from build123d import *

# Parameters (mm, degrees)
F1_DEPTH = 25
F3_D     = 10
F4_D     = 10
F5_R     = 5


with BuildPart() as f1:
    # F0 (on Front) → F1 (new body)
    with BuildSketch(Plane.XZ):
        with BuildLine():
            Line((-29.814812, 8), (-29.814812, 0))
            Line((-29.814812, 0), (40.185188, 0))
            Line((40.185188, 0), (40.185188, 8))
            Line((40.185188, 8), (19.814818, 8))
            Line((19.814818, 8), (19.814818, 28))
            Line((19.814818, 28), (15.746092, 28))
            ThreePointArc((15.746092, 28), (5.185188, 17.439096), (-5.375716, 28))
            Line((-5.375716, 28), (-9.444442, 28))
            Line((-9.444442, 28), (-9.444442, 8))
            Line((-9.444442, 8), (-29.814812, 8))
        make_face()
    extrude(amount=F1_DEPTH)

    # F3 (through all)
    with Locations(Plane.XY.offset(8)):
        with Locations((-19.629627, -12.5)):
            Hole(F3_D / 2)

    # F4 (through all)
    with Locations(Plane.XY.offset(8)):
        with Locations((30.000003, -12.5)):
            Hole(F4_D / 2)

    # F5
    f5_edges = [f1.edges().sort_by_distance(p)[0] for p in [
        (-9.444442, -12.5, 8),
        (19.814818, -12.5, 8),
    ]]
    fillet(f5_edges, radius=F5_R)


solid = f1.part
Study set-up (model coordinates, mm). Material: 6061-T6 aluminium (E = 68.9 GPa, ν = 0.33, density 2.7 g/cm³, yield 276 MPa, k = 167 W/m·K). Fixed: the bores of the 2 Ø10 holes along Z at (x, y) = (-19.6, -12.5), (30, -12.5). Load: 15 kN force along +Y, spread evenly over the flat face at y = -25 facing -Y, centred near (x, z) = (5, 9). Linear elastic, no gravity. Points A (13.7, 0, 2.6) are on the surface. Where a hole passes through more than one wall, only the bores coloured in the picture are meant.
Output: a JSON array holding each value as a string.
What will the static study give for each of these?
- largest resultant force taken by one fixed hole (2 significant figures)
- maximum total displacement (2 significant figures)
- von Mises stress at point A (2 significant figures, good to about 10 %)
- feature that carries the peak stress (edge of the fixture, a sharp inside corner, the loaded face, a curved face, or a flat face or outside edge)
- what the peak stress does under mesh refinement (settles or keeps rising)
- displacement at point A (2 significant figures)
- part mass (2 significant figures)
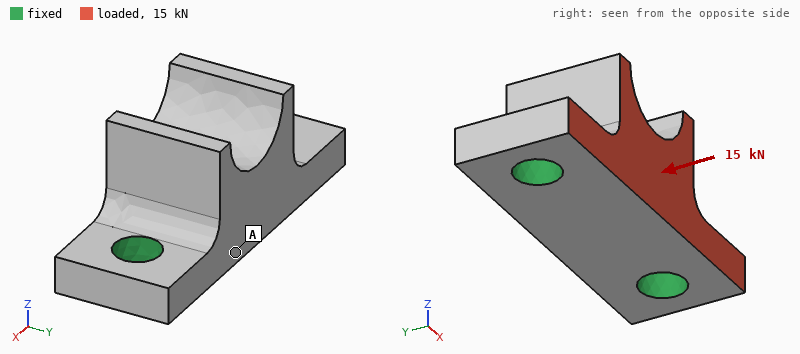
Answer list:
["7.5 kN", "86 µm", "38 MPa", "edge of the fixture", "keeps rising", "31 µm", "63 g"]
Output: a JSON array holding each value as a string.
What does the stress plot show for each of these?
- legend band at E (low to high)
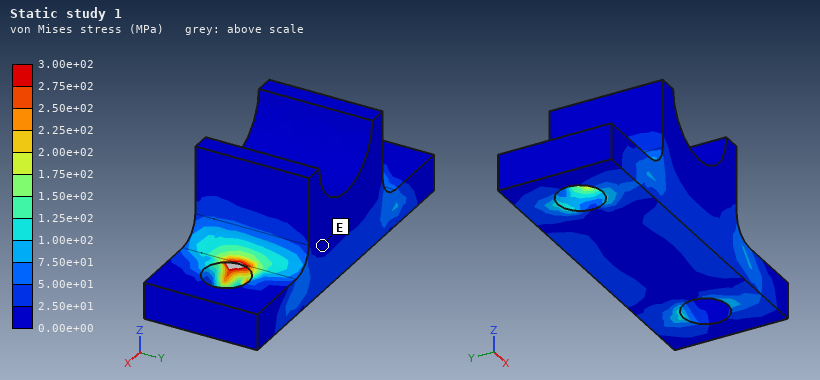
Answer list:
["0.00e+00 to 2.50e+01 MPa"]
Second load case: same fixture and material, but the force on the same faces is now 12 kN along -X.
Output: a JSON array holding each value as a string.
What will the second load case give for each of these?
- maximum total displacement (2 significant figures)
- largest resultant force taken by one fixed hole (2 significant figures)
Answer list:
["34 µm", "6.7 kN"]
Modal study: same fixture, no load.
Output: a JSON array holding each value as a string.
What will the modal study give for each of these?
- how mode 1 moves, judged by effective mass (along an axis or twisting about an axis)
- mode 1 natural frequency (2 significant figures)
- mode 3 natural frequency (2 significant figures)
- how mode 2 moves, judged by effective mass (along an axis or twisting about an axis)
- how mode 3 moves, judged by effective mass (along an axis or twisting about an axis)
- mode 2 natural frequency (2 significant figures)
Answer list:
["along Y", "9800 Hz", "23 kHz", "along Z", "along X", "17 kHz"]
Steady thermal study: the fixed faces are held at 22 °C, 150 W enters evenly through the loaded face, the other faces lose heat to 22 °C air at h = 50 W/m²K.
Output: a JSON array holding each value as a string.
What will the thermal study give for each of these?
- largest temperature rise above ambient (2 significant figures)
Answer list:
["30 K"]
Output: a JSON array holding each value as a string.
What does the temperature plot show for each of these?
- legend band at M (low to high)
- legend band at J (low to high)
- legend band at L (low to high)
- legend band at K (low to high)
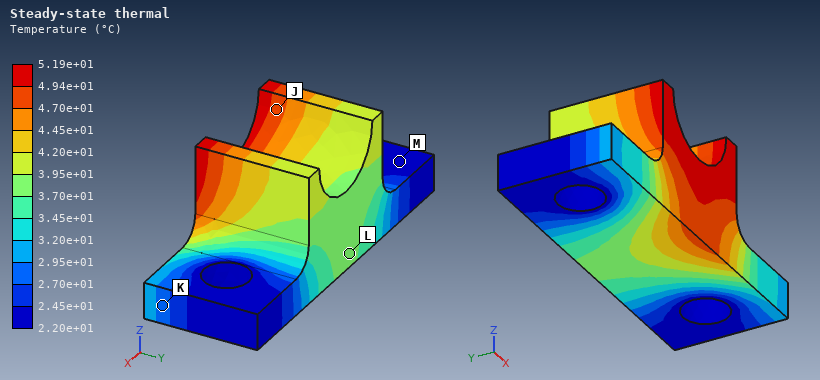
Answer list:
["2.20e+01 to 2.45e+01 °C", "4.70e+01 to 4.94e+01 °C", "3.70e+01 to 3.95e+01 °C", "2.70e+01 to 2.95e+01 °C"]
